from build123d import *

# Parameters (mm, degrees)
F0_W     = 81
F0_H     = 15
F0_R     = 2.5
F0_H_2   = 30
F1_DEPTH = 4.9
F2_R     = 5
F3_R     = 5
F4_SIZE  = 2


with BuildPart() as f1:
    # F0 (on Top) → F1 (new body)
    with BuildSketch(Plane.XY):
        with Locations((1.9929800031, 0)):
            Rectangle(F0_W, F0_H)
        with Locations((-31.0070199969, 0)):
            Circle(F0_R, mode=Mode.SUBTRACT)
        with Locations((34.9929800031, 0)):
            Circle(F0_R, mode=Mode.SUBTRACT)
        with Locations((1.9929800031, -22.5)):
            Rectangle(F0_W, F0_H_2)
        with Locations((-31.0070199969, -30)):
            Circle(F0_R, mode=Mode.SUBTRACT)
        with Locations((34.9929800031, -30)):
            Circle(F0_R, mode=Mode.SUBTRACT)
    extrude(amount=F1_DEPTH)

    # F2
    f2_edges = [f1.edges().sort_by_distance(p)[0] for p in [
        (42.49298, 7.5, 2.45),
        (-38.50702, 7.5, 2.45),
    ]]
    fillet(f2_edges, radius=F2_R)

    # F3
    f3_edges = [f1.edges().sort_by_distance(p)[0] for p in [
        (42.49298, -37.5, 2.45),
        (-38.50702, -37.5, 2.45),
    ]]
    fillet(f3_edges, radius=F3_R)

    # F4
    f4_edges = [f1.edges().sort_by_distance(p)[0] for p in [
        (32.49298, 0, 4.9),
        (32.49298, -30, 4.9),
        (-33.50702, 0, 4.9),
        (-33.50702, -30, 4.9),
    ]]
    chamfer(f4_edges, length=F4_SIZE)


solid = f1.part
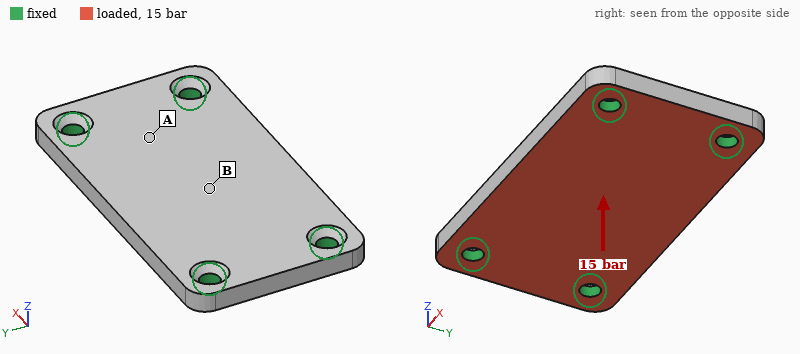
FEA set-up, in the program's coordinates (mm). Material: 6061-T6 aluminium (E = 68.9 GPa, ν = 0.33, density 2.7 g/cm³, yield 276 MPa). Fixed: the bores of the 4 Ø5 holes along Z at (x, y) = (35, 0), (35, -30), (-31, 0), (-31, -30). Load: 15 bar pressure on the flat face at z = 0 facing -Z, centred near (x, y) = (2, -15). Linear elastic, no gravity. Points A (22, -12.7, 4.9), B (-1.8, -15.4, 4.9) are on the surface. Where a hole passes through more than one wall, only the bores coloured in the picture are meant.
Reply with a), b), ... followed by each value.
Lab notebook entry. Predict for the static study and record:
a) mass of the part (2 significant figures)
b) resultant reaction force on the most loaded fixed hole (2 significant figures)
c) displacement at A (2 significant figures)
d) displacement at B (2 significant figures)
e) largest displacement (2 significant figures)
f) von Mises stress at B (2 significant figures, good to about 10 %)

a) 46 g
b) 1.5 kN
c) 0.076 mm
d) 0.14 mm
e) 0.16 mm
f) 72 MPa
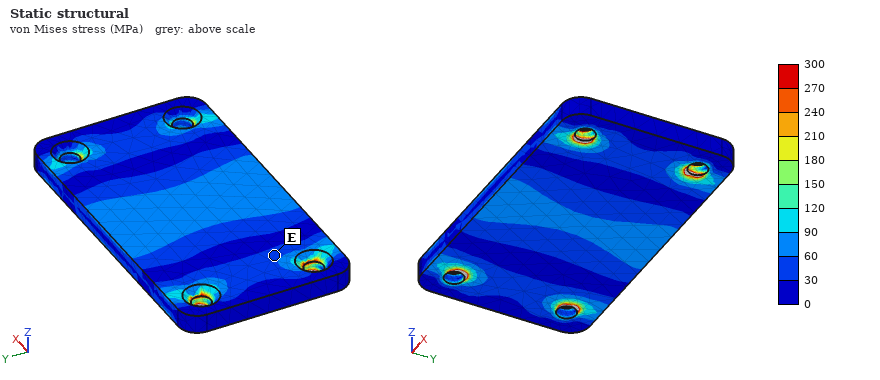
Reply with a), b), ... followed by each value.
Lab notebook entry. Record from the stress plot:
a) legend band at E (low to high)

a) 30 to 60 MPa
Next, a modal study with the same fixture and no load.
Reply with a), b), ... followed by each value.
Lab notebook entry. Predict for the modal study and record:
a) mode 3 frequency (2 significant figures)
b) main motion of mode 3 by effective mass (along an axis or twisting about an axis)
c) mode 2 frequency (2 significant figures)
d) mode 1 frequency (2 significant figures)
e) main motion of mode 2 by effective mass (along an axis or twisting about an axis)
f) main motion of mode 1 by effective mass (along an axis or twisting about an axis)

a) 13 kHz
b) twisting about Y
c) 7300 Hz
d) 4900 Hz
e) twisting about X
f) along Z
